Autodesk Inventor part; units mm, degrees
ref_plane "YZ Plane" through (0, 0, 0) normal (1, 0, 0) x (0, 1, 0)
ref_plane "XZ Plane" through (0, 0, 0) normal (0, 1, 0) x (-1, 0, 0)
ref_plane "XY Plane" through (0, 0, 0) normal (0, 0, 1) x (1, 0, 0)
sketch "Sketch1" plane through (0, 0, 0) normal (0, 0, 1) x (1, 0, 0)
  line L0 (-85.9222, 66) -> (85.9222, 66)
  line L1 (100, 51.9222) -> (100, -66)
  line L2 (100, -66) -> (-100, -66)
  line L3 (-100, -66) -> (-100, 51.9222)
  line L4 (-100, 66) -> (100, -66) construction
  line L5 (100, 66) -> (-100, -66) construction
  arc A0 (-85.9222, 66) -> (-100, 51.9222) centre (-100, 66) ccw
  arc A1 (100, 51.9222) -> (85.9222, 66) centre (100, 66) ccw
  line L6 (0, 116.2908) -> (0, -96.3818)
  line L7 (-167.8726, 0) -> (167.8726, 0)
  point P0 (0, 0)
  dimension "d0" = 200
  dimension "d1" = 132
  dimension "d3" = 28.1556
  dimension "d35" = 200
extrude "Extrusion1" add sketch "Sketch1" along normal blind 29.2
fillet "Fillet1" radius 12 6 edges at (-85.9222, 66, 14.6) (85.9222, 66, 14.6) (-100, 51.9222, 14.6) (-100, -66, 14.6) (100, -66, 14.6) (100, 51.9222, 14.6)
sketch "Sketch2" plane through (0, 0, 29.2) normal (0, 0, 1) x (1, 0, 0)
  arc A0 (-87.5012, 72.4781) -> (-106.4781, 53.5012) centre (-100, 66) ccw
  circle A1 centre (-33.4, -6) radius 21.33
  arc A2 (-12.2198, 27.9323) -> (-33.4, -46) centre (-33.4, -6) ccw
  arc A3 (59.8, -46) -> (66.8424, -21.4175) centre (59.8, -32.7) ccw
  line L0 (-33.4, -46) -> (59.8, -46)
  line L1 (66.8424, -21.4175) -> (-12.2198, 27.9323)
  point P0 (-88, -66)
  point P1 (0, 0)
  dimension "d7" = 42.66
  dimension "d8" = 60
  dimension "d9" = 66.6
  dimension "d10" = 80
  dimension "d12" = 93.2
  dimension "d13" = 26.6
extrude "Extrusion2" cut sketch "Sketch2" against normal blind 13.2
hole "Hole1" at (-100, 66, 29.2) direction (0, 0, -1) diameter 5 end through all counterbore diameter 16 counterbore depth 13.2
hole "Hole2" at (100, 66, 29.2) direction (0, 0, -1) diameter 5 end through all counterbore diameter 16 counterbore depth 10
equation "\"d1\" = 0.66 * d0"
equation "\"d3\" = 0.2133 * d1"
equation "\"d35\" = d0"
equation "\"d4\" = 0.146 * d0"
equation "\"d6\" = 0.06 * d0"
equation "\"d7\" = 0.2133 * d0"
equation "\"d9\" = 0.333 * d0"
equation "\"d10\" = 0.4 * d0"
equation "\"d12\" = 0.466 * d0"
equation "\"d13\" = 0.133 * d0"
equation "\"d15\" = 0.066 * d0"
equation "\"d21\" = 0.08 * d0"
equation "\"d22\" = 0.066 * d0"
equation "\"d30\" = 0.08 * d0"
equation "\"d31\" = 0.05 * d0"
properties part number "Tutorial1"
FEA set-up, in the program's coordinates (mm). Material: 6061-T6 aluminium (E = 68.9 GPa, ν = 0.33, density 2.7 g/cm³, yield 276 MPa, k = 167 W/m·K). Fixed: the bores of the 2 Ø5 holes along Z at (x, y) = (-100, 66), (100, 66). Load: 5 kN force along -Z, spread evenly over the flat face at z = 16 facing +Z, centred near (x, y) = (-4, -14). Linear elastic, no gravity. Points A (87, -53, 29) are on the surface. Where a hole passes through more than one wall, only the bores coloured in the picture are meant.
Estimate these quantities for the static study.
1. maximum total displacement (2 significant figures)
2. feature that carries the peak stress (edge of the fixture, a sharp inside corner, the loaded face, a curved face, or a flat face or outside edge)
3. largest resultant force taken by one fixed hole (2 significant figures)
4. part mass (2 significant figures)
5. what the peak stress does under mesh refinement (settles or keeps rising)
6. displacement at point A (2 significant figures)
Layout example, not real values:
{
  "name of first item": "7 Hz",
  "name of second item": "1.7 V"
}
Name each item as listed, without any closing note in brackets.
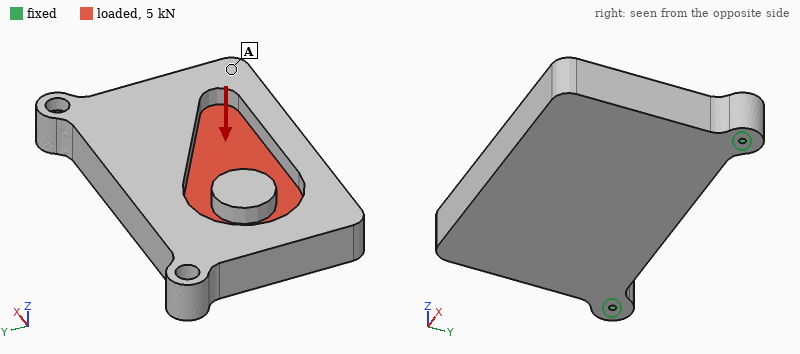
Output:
{
  "maximum total displacement": "0.56 mm",
  "feature that carries the peak stress": "edge of the fixture",
  "largest resultant force taken by one fixed hole": "2.7 kN",
  "part mass": "1.9 kg",
  "what the peak stress does under mesh refinement": "keeps rising",
  "displacement at point A": "0.46 mm"
}
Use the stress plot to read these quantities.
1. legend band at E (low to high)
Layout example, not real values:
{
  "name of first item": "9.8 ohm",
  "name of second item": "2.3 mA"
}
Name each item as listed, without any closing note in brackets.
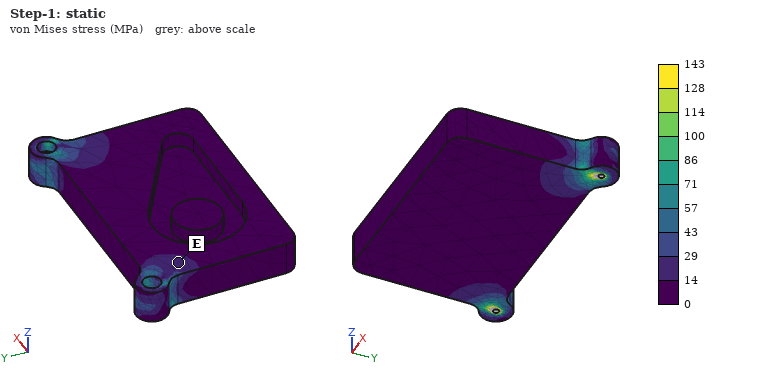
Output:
{
  "legend band at E": "14 to 29 MPa"
}
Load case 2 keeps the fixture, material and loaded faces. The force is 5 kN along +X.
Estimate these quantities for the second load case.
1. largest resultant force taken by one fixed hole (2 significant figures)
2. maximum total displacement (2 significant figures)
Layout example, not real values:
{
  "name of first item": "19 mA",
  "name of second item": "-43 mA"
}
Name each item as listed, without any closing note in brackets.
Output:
{
  "largest resultant force taken by one fixed hole": "3.2 kN",
  "maximum total displacement": "13 µm"
}
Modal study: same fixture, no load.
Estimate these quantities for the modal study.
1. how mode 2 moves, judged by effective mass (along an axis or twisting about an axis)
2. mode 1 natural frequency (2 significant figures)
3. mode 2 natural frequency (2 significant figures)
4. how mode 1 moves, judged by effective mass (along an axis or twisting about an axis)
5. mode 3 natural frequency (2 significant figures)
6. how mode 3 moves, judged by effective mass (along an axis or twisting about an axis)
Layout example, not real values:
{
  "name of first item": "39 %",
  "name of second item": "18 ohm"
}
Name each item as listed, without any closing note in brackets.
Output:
{
  "how mode 2 moves, judged by effective mass": "twisting about Y",
  "mode 1 natural frequency": "490 Hz",
  "mode 2 natural frequency": "1500 Hz",
  "how mode 1 moves, judged by effective mass": "along Z",
  "mode 3 natural frequency": "2400 Hz",
  "how mode 3 moves, judged by effective mass": "along Z"
}
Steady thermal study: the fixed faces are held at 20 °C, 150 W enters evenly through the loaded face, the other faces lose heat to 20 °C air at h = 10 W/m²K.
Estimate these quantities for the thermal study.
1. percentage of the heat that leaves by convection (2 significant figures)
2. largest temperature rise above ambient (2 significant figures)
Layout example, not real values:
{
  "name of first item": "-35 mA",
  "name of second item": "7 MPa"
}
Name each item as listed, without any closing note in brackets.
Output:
{
  "percentage of the heat that leaves by convection": "12 %",
  "largest temperature rise above ambient": "34 K"
}
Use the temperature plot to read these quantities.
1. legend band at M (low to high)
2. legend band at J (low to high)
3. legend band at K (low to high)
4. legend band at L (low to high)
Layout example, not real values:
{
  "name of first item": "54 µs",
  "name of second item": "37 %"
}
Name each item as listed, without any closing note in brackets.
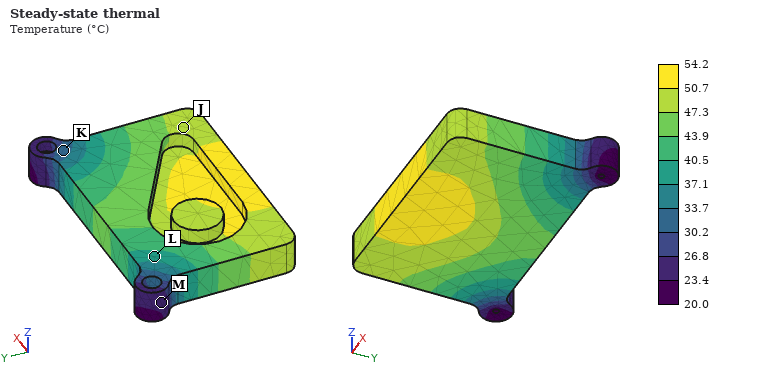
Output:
{
  "legend band at M": "23.4 to 26.8 °C",
  "legend band at J": "47.3 to 50.7 °C",
  "legend band at K": "30.2 to 33.7 °C",
  "legend band at L": "37.1 to 40.5 °C"
}
